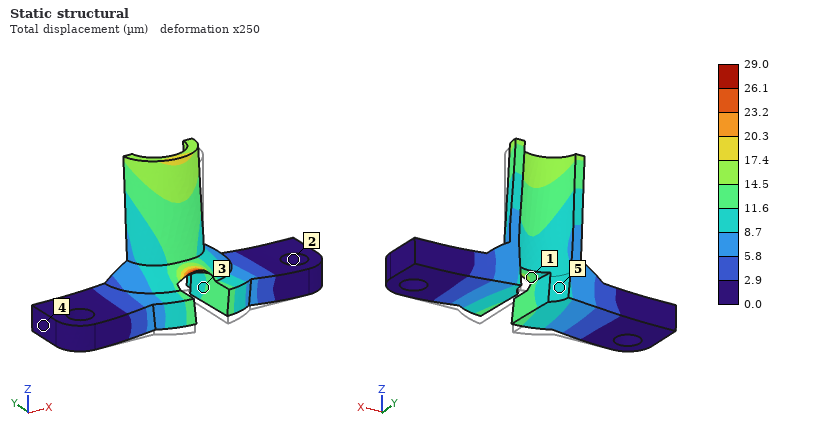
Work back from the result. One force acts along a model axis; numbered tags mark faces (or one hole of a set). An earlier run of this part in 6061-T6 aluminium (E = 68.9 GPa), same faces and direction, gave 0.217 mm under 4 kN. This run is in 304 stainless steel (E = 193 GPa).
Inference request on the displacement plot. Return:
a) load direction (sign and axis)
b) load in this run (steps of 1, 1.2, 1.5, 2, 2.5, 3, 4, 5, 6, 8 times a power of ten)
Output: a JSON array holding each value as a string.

["+Z", "1.5 kN"]
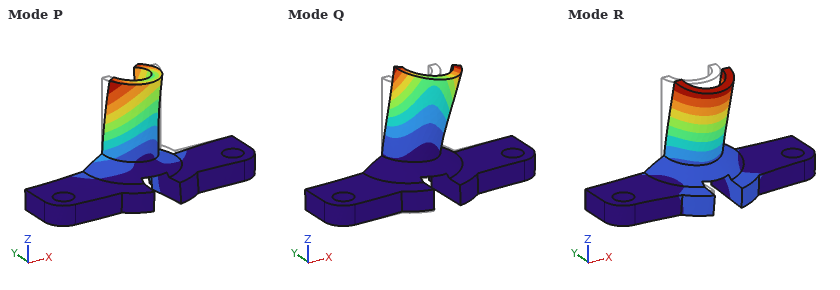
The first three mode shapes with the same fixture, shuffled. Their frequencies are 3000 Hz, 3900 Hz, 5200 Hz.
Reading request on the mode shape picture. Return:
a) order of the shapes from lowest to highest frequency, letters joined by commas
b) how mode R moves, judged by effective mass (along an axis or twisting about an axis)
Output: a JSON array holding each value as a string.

["R, Q, P", "along Y"]
